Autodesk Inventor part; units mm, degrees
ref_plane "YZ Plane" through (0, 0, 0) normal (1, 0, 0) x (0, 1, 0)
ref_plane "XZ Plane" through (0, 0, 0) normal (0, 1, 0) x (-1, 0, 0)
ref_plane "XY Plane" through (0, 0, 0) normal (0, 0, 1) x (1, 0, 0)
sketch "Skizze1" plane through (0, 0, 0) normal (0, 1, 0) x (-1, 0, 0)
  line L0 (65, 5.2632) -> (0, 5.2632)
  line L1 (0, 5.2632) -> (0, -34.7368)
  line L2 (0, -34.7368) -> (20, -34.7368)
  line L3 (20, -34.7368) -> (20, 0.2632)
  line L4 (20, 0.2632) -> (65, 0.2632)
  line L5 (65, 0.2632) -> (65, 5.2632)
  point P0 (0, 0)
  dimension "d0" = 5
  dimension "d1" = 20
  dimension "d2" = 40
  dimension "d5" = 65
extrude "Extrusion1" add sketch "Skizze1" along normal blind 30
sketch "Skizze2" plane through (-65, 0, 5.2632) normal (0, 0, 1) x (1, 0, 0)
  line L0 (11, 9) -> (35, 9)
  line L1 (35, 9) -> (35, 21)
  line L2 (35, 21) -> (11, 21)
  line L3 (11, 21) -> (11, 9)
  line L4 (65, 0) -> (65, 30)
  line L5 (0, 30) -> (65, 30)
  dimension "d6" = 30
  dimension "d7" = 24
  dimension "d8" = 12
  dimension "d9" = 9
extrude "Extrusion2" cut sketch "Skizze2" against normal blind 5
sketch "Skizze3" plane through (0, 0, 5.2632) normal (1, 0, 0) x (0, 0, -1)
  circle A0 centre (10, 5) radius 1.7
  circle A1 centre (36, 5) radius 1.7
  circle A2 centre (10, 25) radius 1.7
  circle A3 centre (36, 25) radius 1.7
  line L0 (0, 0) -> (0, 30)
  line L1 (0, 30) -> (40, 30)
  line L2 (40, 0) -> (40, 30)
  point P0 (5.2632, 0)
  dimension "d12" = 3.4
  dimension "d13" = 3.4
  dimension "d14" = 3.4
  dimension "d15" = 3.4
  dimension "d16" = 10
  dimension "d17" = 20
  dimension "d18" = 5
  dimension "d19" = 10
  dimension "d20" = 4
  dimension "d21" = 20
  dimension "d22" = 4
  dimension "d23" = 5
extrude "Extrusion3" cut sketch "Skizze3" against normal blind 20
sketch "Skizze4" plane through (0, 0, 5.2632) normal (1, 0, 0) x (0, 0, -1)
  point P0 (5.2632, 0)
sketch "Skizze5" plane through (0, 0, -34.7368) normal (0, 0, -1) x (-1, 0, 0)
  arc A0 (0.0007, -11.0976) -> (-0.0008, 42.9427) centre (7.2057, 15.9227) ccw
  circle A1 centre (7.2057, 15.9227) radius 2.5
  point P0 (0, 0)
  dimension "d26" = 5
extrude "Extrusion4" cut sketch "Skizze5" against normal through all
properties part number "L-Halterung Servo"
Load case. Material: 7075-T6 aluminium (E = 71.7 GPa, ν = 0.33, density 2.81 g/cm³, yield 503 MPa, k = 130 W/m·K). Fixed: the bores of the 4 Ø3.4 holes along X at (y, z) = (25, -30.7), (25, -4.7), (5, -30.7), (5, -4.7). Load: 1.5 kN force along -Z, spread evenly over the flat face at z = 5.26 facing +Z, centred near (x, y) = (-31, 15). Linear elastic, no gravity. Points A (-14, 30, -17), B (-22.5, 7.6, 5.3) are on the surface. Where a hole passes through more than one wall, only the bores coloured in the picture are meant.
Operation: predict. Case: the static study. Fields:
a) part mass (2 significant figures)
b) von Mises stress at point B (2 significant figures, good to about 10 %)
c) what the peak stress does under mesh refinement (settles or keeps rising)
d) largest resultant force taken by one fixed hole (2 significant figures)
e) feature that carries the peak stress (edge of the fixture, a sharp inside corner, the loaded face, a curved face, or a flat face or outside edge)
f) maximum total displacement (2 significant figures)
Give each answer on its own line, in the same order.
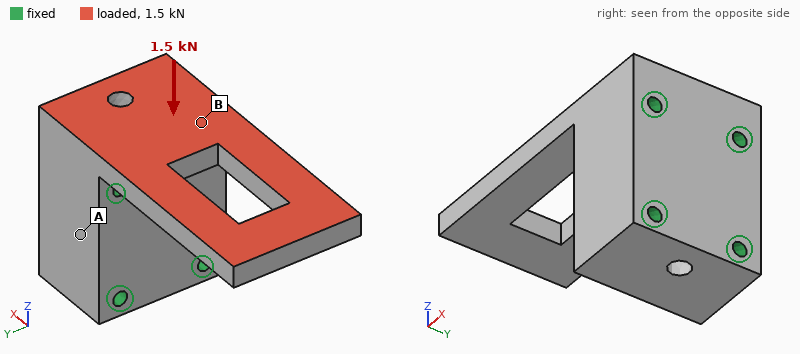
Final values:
78 g
140 MPa
keeps rising
690 N
a sharp inside corner
0.83 mm
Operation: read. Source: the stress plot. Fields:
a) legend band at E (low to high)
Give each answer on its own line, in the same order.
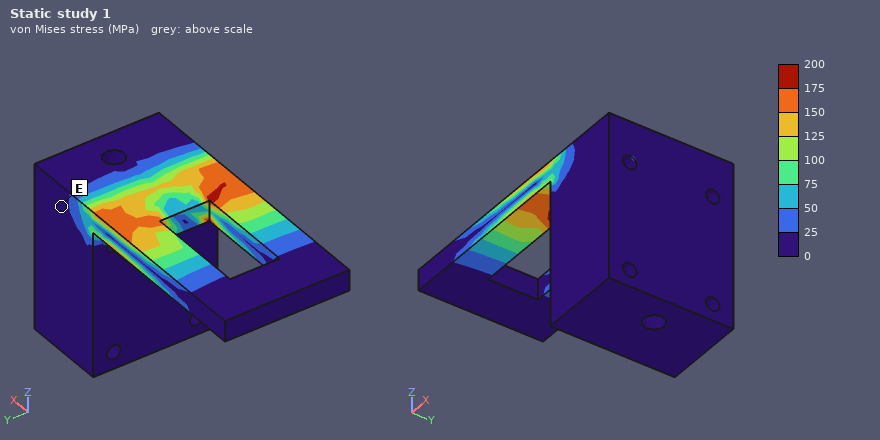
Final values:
0 to 25 MPa
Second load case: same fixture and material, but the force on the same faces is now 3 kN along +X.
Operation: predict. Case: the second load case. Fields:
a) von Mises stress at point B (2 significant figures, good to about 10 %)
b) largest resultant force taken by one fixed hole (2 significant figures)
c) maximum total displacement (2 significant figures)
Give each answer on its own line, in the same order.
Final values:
46 MPa
1.6 kN
0.25 mm
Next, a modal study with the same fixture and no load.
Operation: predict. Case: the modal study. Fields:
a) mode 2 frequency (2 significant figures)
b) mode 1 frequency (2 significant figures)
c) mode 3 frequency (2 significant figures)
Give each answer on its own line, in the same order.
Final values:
4900 Hz
1700 Hz
5400 Hz
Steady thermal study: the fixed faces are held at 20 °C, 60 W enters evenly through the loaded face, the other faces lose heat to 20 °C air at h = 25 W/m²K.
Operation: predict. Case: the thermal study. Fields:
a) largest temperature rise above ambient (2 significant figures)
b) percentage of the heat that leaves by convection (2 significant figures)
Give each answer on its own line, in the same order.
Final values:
73 K
4.5 %
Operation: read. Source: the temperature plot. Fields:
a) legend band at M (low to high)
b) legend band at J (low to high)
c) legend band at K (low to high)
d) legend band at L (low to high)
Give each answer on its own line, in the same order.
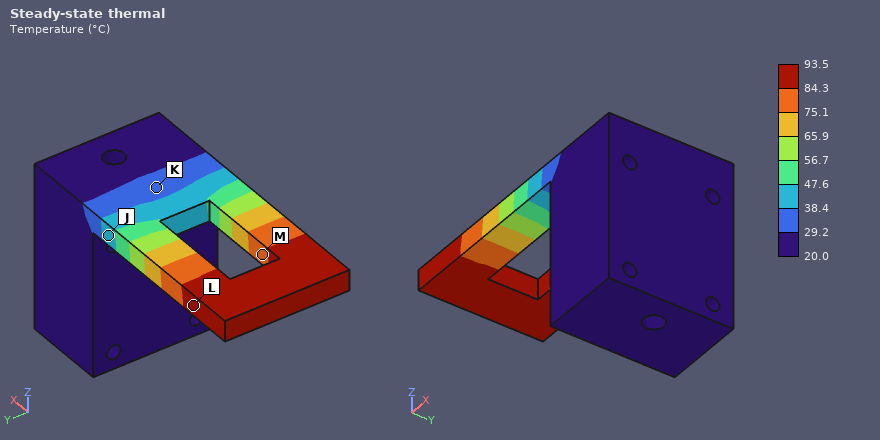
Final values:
75.1 to 84.3 °C
38.4 to 47.6 °C
29.2 to 38.4 °C
84.3 to 93.5 °C
